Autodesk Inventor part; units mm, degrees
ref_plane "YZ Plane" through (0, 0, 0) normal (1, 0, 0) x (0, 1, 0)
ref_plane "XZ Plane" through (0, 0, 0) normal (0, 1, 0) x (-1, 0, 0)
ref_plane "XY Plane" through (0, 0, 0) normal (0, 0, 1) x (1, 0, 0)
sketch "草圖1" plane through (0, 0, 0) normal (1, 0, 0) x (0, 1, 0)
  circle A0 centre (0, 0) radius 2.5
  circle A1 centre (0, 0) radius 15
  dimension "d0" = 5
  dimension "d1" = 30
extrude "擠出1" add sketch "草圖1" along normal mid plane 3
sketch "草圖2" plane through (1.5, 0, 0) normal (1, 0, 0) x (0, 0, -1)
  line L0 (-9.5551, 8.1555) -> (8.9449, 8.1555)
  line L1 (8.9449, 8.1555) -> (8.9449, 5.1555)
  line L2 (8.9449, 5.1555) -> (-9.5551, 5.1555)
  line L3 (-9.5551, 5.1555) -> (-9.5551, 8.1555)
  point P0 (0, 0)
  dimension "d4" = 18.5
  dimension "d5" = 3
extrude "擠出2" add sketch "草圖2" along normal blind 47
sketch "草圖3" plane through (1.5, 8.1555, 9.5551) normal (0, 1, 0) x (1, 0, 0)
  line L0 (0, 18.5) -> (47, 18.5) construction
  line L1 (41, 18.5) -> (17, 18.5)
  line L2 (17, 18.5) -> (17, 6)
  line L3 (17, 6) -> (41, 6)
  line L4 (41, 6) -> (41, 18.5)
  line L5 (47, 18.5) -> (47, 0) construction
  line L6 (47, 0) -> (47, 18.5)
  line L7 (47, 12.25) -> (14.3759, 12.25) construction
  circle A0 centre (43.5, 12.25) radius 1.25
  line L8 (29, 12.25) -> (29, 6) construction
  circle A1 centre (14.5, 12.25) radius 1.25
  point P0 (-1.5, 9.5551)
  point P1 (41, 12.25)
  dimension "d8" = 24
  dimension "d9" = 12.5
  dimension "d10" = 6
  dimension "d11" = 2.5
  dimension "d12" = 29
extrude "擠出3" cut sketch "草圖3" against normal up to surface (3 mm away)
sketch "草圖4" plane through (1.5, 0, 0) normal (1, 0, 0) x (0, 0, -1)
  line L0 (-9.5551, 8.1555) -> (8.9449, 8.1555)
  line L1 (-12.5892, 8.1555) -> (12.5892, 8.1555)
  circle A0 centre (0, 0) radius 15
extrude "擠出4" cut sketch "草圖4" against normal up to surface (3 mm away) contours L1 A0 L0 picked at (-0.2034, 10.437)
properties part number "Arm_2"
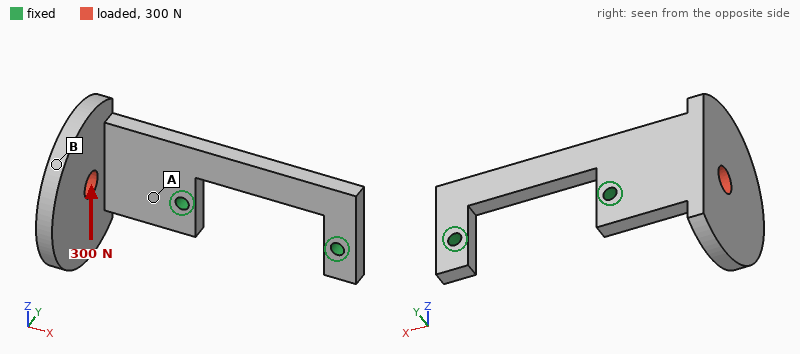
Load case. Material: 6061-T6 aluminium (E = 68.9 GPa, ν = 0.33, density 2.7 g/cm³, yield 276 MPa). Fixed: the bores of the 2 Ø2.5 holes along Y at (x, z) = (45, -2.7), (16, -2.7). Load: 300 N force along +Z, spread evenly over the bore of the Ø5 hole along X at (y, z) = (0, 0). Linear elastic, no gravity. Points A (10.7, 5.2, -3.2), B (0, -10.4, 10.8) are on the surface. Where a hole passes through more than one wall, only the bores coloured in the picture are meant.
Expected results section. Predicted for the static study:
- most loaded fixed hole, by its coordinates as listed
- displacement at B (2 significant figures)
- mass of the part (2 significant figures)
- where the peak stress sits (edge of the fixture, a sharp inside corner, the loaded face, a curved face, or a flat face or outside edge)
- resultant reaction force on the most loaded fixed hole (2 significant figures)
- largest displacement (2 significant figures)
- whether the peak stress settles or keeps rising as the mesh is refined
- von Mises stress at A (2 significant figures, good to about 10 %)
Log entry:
(16, -2.7)
0.20 mm
9.1 g
edge of the fixture
400 N
0.21 mm
keeps rising
84 MPa
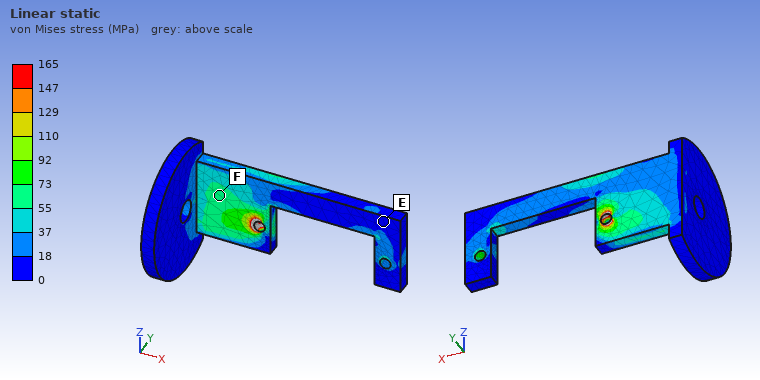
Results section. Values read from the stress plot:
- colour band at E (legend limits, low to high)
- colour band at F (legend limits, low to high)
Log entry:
0 to 18 MPa
55 to 73 MPa
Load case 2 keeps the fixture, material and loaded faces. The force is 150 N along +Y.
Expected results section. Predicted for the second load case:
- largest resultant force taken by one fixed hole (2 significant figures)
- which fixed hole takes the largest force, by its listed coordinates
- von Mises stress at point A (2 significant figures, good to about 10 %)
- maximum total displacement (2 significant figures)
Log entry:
160 N
(16, -2.7)
63 MPa
0.20 mm
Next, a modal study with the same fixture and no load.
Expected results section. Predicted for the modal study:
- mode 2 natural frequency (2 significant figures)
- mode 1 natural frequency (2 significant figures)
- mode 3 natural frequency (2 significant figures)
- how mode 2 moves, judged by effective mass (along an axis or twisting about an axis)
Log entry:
2600 Hz
2000 Hz
5900 Hz
along Z
